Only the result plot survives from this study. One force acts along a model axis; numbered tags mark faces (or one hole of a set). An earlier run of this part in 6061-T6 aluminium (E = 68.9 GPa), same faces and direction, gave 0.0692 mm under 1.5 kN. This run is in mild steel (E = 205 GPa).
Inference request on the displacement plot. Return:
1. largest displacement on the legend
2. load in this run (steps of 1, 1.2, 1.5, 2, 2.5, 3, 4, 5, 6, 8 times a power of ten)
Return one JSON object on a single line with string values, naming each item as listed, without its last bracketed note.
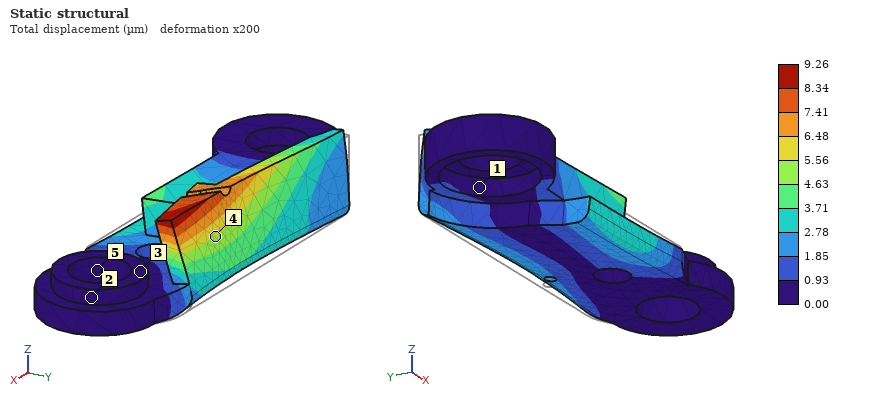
{"largest displacement on the legend": "9.26 µm", "load in this run": "600 N"}
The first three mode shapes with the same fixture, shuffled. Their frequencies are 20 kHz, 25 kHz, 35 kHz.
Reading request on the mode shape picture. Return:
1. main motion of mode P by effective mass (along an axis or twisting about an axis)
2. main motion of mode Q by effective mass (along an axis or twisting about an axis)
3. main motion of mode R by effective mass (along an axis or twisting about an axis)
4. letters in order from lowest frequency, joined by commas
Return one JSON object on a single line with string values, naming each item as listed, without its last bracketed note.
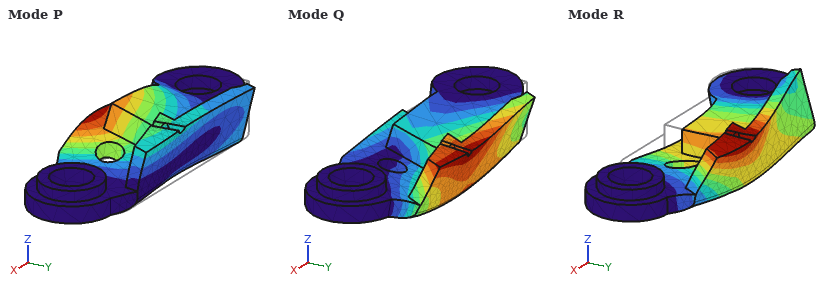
{"main motion of mode P by effective mass": "along Z", "main motion of mode Q by effective mass": "along Z", "main motion of mode R by effective mass": "along Y", "letters in order from lowest frequency, joined by commas": "Q, P, R"}
